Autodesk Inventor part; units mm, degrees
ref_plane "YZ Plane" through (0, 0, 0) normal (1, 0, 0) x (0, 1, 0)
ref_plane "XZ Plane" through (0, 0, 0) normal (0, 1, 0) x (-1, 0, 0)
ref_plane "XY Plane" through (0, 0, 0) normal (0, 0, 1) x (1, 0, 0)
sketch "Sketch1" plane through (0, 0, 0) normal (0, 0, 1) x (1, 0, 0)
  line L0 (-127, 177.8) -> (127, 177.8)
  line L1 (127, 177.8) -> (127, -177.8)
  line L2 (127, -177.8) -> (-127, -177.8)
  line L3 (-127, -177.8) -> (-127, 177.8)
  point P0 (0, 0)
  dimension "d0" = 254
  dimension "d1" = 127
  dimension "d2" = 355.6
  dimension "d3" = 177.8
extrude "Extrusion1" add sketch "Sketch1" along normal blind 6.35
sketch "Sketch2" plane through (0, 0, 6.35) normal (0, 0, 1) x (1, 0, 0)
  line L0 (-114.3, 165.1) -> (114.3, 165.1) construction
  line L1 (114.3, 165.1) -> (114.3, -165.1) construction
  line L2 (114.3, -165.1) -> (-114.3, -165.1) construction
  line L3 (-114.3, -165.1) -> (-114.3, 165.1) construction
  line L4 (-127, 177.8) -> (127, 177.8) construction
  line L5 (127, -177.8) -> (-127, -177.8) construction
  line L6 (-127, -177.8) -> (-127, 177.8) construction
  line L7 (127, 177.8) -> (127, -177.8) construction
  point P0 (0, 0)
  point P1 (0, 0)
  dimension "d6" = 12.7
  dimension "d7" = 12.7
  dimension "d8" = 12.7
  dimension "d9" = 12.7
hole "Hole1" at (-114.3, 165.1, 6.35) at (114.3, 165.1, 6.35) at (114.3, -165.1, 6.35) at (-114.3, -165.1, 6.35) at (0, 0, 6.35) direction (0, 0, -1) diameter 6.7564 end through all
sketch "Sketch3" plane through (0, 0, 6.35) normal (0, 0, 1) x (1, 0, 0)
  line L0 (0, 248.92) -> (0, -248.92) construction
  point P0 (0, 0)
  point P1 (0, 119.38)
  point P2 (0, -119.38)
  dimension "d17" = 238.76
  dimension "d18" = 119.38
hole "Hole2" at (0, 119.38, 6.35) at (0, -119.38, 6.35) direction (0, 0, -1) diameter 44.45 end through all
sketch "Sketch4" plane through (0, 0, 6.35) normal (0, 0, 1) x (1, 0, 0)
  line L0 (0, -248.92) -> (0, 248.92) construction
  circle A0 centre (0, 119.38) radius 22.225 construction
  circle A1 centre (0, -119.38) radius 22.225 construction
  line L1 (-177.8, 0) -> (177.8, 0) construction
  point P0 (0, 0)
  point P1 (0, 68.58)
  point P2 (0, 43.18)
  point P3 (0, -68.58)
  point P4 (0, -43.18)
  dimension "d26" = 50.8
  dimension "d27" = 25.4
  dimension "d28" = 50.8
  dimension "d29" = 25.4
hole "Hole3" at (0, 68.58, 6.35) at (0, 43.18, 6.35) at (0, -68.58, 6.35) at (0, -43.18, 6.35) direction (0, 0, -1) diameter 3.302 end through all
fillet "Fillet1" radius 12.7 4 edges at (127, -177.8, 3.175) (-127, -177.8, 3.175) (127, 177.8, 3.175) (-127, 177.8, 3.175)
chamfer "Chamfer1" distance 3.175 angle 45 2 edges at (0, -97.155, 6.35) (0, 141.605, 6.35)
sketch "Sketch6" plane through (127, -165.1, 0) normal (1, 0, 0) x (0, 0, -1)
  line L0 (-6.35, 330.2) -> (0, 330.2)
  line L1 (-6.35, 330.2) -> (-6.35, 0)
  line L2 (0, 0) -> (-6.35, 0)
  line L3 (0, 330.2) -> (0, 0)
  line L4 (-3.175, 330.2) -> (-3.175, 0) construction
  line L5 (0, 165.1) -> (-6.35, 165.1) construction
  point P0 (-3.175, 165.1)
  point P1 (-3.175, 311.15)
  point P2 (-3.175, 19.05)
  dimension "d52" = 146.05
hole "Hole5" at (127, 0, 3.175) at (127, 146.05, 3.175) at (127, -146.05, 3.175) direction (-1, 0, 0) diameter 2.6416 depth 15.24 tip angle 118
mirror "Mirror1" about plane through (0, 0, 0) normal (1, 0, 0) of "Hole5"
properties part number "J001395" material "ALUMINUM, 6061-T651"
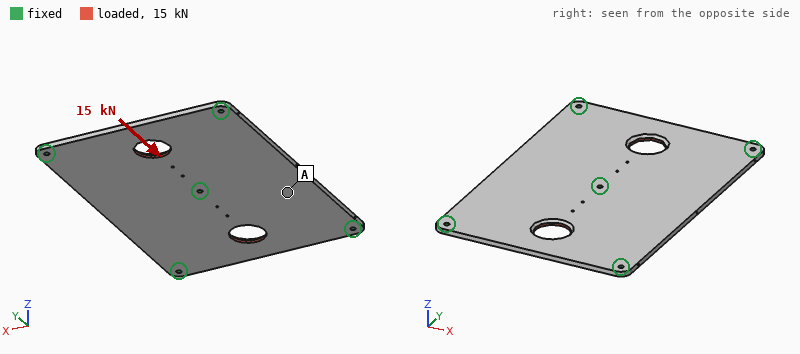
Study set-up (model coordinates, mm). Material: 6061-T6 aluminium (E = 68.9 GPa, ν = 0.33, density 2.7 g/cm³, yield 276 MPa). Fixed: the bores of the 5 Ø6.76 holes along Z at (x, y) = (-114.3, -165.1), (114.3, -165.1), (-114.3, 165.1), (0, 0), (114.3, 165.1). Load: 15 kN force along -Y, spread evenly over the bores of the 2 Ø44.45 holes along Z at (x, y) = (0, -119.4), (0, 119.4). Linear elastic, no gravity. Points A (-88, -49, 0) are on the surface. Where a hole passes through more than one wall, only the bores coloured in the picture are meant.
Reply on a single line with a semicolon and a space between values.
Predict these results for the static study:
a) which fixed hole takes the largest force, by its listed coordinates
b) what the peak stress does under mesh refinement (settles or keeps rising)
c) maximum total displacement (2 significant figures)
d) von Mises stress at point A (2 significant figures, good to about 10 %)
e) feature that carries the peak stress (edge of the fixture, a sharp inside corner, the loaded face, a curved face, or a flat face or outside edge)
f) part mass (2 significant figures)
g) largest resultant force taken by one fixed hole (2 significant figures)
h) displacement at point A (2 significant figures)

(0, 0); keeps rising; 81 µm; 3.2 MPa; edge of the fixture; 1.5 kg; 6.5 kN; 15 µm
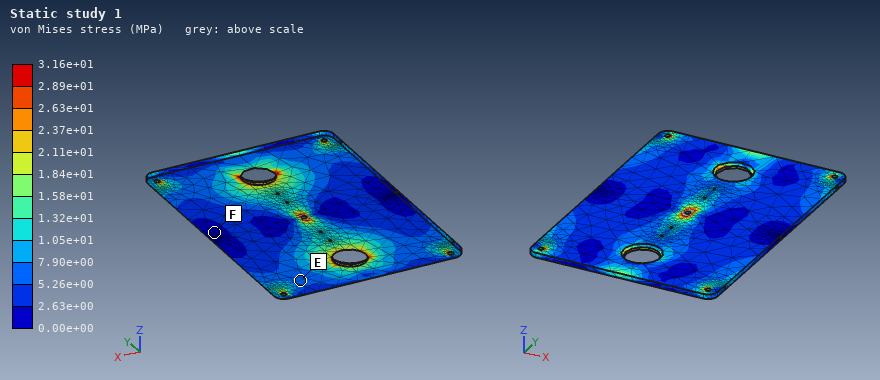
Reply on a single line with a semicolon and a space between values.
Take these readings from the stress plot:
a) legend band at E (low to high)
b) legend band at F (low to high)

5.26e+00 to 7.90e+00 MPa; 0.00e+00 to 2.63e+00 MPa
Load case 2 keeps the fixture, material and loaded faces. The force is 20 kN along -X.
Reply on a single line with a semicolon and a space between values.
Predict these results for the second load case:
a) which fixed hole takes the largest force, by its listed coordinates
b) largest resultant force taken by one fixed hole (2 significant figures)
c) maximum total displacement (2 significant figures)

(0, 0); 6.2 kN; 39 µm
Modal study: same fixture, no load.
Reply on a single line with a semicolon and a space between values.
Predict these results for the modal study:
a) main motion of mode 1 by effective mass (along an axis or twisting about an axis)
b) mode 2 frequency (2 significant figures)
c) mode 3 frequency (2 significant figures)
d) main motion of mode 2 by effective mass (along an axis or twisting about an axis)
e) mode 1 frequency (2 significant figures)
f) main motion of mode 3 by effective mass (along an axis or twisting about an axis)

twisting about Y; 500 Hz; 590 Hz; along Z; 440 Hz; twisting about X
